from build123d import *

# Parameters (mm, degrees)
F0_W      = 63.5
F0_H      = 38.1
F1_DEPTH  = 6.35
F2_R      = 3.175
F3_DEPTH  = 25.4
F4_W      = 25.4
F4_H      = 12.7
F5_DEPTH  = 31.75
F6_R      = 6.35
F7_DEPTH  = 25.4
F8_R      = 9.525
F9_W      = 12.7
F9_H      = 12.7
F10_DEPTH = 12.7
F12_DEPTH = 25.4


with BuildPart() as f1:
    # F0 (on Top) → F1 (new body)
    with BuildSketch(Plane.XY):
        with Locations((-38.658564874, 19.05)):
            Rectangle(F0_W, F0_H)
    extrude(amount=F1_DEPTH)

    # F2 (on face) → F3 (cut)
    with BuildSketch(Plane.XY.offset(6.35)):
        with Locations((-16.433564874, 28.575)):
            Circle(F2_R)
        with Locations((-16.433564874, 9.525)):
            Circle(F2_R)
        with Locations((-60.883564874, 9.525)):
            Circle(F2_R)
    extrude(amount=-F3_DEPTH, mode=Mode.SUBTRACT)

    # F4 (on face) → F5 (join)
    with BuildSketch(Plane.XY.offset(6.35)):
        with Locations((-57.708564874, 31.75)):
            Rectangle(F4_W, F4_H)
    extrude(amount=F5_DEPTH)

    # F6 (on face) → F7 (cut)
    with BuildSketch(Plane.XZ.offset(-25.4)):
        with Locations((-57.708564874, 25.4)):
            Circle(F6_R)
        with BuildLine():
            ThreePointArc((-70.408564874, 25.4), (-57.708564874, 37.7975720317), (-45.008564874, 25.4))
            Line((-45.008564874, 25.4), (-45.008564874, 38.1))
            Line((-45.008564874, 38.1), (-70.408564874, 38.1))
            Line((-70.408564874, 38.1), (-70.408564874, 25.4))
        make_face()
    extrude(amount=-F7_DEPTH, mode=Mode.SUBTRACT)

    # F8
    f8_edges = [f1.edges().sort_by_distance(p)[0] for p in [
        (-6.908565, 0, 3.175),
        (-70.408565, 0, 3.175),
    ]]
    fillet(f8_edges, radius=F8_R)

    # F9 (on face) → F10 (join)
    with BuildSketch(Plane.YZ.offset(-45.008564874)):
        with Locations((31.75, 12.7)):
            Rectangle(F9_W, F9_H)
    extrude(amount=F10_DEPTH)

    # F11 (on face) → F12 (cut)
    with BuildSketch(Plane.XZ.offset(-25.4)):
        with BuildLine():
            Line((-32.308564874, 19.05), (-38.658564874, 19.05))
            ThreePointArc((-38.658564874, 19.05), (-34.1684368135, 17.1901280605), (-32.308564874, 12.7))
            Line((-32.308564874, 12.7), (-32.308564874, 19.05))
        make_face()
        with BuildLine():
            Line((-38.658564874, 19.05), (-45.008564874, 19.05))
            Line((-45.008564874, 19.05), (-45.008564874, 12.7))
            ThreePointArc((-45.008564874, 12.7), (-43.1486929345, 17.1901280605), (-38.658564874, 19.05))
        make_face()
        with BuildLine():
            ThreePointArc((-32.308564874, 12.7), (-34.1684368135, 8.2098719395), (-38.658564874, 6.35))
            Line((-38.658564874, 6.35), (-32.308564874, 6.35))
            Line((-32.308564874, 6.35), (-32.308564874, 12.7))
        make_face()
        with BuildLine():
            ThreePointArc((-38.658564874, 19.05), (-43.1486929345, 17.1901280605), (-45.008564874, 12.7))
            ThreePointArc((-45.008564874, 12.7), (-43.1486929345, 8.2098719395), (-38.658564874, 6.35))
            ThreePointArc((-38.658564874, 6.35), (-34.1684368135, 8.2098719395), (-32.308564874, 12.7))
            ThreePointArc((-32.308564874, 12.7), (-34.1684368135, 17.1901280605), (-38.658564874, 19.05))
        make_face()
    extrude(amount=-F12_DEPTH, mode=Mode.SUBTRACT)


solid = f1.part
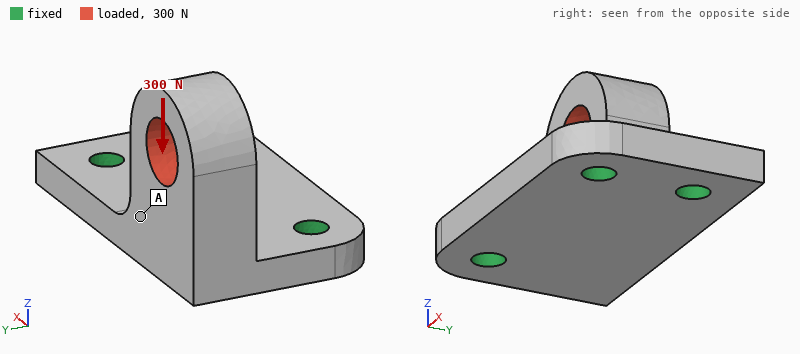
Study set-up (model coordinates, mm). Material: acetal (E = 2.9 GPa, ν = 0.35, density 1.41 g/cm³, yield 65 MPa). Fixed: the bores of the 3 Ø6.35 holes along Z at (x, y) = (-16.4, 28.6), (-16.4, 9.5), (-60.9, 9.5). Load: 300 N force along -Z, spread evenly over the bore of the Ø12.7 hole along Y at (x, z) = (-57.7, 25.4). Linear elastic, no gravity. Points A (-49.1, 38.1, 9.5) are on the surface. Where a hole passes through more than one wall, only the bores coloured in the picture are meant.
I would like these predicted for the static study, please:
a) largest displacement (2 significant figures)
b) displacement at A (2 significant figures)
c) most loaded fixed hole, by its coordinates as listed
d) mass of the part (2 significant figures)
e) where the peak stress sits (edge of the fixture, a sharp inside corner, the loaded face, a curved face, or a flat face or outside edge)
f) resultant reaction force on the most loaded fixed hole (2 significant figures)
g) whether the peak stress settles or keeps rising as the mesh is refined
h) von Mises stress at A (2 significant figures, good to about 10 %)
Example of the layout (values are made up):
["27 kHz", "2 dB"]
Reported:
["0.85 mm", "0.41 mm", "(-60.9, 9.5)", "31 g", "edge of the fixture", "240 N", "keeps rising", "3.1 MPa"]
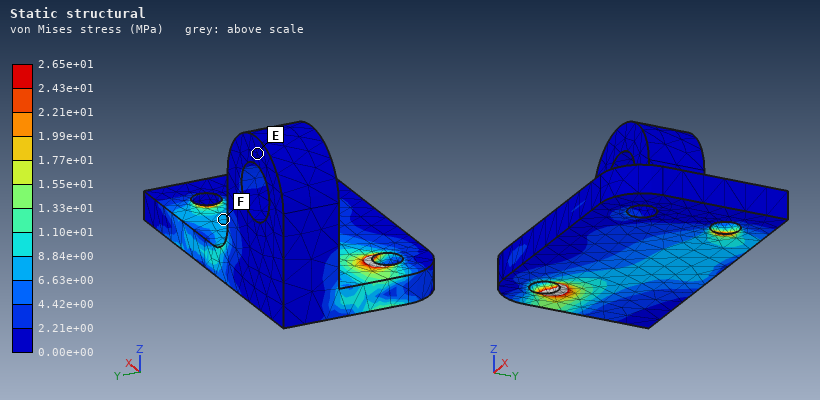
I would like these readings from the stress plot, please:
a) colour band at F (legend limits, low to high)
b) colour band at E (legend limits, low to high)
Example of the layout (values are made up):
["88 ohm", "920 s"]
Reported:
["6.63e+00 to 8.84e+00 MPa", "0.00e+00 to 2.21e+00 MPa"]
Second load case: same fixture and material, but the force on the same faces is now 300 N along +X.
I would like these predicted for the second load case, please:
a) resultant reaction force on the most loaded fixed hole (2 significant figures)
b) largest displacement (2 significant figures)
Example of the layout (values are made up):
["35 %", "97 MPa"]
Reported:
["190 N", "0.62 mm"]
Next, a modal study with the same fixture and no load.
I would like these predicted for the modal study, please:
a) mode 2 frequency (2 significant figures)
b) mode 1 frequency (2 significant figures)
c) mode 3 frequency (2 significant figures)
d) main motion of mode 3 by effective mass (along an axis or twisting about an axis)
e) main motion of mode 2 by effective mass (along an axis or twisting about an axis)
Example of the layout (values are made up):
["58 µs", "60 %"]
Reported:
["1600 Hz", "810 Hz", "2500 Hz", "along Z", "along X"]
